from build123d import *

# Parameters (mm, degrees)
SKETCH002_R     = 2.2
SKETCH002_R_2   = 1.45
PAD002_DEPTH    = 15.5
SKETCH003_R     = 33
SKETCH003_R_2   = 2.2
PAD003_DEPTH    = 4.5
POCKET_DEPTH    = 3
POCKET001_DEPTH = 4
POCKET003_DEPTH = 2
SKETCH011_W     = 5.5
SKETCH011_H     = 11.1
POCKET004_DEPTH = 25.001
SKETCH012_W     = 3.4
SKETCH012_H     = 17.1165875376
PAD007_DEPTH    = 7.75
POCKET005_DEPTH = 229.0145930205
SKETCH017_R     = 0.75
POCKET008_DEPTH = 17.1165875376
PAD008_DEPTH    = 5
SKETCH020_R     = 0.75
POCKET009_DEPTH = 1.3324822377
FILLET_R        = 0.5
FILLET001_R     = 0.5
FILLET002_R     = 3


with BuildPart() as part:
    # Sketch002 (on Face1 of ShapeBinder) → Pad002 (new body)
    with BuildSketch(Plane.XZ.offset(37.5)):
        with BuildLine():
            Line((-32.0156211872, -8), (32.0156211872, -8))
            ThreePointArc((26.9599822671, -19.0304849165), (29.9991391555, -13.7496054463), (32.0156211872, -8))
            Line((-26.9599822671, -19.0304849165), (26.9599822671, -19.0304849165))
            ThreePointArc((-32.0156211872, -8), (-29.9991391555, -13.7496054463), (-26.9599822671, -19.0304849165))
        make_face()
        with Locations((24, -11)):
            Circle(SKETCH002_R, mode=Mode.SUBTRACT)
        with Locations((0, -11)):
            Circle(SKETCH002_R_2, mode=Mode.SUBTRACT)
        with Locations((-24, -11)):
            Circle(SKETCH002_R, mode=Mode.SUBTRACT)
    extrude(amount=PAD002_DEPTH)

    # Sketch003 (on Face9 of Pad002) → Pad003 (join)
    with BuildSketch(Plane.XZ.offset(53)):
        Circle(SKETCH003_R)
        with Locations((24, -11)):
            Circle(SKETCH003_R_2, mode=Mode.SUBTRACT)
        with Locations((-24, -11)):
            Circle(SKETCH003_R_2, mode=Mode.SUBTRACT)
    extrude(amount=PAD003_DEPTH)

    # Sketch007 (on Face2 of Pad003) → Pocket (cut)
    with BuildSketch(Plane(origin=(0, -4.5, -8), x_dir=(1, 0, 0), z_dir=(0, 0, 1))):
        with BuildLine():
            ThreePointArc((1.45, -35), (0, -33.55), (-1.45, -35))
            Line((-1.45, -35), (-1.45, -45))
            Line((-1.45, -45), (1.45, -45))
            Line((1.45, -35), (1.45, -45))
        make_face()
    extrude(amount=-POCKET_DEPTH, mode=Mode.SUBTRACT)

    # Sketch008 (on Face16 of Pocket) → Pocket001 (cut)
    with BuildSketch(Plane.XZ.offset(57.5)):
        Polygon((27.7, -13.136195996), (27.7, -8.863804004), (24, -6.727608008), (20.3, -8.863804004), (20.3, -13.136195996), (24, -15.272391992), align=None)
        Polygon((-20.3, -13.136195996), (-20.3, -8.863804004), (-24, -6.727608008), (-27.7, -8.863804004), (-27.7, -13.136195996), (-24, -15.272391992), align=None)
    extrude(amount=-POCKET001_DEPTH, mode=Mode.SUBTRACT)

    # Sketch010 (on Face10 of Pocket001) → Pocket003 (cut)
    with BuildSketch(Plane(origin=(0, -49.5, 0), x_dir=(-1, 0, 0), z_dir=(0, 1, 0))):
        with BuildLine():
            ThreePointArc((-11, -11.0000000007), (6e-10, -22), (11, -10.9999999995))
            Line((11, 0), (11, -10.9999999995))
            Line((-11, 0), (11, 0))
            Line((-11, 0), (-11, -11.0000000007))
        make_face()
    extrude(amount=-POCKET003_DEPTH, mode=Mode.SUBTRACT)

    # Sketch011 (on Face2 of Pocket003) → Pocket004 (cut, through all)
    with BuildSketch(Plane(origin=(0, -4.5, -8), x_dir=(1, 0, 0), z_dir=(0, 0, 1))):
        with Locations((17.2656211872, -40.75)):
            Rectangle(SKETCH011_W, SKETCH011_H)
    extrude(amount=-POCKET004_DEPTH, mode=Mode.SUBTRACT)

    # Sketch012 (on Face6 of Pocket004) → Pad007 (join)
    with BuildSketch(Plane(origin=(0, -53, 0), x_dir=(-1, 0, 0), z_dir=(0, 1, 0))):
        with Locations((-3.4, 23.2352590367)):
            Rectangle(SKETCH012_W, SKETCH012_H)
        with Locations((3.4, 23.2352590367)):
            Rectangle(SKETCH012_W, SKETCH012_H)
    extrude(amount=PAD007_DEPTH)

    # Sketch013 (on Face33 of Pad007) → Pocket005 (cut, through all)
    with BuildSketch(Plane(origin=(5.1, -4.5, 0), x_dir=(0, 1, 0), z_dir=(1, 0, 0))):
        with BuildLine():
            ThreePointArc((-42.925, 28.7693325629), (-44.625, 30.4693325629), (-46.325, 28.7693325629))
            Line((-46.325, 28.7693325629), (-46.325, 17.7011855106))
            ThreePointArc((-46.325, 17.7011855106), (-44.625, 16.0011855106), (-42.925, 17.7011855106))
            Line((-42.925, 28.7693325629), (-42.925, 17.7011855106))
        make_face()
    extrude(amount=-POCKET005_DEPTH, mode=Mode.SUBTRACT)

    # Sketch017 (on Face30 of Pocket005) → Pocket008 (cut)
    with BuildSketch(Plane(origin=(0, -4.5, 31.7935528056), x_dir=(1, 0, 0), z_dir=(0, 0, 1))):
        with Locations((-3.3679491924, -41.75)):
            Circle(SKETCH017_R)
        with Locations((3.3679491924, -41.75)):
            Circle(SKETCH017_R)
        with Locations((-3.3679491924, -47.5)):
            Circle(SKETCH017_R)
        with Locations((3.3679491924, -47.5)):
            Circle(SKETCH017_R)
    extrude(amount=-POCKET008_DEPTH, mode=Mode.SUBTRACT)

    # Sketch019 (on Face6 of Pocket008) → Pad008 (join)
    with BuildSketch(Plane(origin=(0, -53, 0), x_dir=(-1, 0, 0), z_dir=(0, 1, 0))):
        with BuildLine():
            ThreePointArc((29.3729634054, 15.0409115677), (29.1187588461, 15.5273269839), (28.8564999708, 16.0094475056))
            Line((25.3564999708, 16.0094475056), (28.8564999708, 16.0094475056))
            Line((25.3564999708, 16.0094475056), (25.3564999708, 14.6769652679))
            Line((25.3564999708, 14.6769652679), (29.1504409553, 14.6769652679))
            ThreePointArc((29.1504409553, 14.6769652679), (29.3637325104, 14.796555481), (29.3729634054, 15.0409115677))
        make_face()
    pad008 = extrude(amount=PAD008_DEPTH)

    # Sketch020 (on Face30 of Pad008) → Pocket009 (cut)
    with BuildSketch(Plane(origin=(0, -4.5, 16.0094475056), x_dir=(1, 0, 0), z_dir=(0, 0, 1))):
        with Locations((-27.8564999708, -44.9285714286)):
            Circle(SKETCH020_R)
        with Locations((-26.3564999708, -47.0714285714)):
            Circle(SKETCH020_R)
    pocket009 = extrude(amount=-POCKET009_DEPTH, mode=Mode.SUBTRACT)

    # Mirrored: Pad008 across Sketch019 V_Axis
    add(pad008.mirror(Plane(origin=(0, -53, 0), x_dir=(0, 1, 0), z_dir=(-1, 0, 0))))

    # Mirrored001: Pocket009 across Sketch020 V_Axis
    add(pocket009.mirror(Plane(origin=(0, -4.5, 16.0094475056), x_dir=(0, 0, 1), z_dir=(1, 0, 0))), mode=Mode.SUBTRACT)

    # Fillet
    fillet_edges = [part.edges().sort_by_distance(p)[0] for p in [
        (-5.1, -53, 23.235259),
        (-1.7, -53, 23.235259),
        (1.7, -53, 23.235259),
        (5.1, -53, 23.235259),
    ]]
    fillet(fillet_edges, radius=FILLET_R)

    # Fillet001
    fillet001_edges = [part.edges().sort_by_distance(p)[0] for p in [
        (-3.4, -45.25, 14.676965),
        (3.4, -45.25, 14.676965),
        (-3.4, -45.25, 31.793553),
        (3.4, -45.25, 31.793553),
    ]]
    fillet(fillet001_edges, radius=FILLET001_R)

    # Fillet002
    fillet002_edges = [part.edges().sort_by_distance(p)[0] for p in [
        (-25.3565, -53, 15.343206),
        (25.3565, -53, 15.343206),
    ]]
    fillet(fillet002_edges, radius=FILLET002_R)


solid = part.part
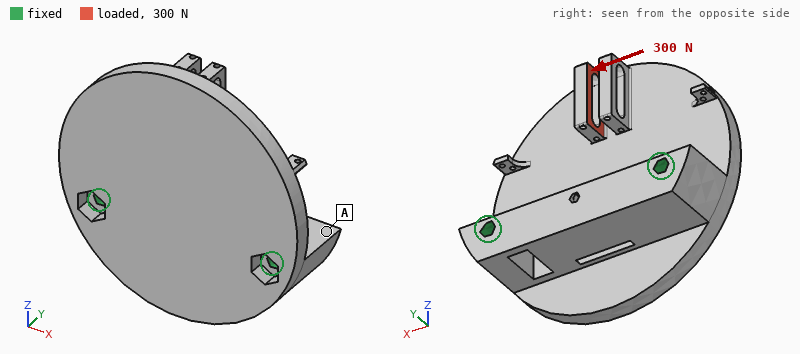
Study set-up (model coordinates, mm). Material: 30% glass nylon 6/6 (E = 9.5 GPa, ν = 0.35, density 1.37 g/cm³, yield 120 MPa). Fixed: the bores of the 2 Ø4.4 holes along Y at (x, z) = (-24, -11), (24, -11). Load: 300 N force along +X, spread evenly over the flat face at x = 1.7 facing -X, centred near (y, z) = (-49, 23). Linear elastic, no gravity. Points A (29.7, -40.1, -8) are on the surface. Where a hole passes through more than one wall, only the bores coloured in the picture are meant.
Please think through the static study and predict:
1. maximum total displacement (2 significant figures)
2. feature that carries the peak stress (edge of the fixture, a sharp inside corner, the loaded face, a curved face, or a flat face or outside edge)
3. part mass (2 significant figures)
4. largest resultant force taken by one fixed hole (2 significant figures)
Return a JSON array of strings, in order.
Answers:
["0.45 mm", "the loaded face", "33 g", "260 N"]
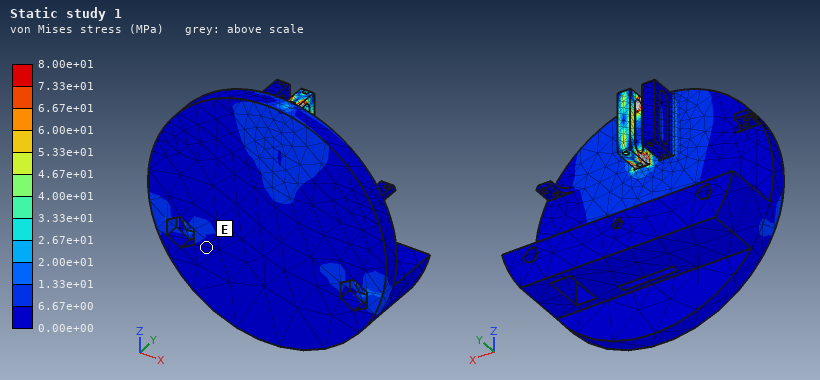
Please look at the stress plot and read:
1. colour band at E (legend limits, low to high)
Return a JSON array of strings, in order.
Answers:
["0.00e+00 to 6.67e+00 MPa"]
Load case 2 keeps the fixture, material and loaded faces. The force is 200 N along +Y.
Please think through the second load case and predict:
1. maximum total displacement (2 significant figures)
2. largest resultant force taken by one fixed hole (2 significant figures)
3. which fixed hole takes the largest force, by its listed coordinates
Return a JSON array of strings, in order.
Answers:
["1.1 mm", "140 N", "(-24, -11)"]
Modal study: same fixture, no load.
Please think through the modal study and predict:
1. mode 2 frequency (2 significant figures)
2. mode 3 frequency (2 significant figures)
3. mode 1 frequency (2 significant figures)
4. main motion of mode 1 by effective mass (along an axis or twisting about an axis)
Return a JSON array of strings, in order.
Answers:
["2600 Hz", "4700 Hz", "1100 Hz", "along Y"]
